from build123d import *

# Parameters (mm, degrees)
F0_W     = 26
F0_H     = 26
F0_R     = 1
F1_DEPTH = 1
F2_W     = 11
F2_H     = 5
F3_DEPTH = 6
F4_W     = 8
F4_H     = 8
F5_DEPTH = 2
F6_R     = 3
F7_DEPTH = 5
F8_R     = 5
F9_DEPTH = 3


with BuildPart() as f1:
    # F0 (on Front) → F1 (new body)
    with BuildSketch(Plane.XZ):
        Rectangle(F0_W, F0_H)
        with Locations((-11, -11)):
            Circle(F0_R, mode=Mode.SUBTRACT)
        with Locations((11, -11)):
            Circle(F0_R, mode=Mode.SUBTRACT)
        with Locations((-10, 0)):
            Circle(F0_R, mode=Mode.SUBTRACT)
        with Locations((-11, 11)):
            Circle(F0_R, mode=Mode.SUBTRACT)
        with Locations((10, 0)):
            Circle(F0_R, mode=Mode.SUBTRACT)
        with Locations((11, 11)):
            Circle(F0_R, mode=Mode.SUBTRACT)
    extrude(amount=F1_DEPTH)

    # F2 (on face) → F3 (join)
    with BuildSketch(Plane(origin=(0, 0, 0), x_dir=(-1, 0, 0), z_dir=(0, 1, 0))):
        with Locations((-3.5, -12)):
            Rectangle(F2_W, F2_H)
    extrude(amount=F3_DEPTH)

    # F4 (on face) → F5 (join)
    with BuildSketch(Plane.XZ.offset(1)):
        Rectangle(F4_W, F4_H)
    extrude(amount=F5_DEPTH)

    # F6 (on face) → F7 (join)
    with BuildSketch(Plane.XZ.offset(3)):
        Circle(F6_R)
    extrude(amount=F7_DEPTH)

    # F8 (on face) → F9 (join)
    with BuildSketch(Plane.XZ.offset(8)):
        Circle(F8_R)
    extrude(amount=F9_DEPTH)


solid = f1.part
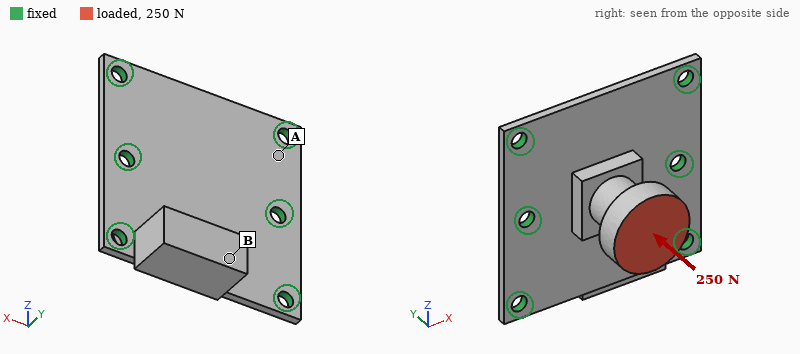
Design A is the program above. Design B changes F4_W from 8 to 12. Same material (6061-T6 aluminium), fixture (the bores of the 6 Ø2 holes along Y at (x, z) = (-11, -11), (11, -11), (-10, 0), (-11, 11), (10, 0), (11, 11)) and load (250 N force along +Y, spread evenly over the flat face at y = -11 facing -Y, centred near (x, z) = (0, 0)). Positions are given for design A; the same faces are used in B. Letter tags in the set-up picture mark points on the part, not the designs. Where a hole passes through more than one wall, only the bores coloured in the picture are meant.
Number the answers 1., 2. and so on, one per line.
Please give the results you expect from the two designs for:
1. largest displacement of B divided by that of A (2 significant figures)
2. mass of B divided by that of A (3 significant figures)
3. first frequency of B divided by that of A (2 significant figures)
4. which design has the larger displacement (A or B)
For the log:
1. 0.54
2. 1.04
3. 1.1
4. A
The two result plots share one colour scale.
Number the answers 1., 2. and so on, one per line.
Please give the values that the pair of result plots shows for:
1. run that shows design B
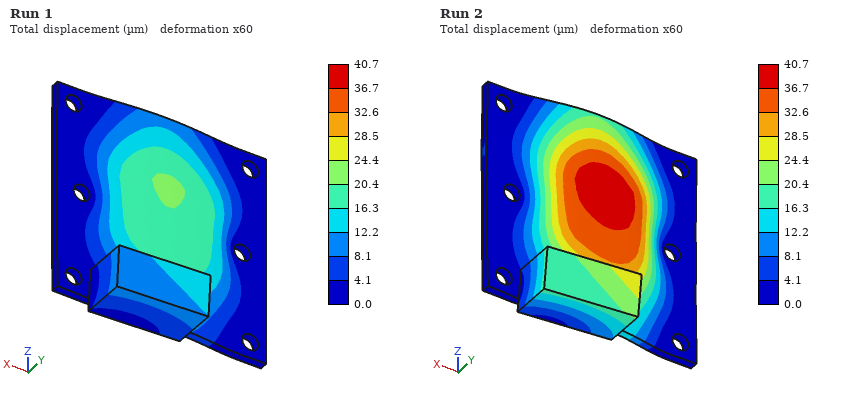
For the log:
1. Run 1
